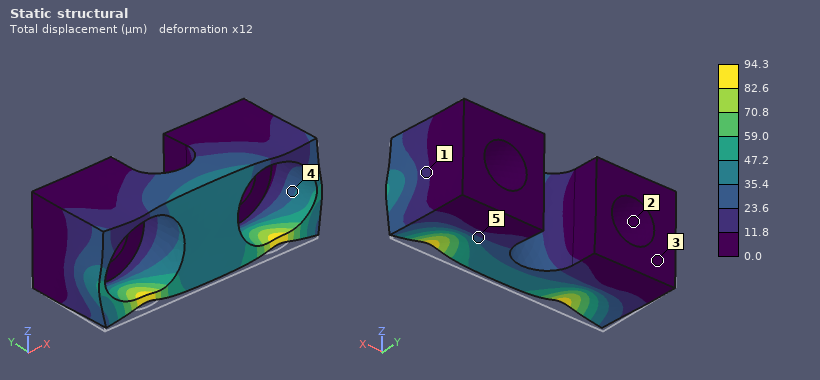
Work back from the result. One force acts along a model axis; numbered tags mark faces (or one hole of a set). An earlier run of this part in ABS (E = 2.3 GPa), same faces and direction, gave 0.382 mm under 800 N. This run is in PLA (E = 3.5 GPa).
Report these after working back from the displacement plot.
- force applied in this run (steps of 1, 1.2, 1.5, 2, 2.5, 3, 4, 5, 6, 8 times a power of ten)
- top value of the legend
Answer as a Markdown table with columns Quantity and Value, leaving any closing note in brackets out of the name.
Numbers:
| Quantity | Value |
|---|---|
| force applied in this run | 300 N |
| top value of the legend | 94.3 µm |
